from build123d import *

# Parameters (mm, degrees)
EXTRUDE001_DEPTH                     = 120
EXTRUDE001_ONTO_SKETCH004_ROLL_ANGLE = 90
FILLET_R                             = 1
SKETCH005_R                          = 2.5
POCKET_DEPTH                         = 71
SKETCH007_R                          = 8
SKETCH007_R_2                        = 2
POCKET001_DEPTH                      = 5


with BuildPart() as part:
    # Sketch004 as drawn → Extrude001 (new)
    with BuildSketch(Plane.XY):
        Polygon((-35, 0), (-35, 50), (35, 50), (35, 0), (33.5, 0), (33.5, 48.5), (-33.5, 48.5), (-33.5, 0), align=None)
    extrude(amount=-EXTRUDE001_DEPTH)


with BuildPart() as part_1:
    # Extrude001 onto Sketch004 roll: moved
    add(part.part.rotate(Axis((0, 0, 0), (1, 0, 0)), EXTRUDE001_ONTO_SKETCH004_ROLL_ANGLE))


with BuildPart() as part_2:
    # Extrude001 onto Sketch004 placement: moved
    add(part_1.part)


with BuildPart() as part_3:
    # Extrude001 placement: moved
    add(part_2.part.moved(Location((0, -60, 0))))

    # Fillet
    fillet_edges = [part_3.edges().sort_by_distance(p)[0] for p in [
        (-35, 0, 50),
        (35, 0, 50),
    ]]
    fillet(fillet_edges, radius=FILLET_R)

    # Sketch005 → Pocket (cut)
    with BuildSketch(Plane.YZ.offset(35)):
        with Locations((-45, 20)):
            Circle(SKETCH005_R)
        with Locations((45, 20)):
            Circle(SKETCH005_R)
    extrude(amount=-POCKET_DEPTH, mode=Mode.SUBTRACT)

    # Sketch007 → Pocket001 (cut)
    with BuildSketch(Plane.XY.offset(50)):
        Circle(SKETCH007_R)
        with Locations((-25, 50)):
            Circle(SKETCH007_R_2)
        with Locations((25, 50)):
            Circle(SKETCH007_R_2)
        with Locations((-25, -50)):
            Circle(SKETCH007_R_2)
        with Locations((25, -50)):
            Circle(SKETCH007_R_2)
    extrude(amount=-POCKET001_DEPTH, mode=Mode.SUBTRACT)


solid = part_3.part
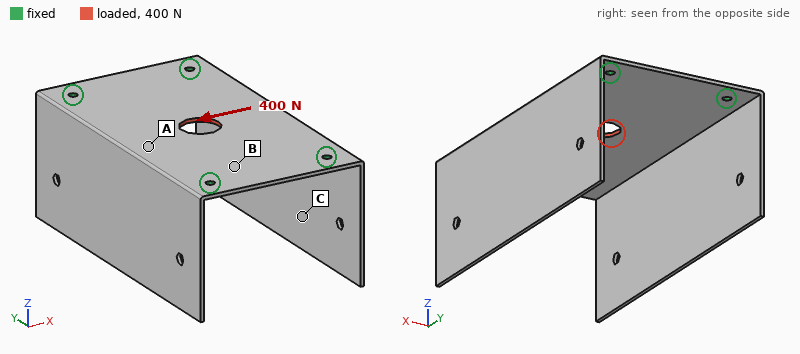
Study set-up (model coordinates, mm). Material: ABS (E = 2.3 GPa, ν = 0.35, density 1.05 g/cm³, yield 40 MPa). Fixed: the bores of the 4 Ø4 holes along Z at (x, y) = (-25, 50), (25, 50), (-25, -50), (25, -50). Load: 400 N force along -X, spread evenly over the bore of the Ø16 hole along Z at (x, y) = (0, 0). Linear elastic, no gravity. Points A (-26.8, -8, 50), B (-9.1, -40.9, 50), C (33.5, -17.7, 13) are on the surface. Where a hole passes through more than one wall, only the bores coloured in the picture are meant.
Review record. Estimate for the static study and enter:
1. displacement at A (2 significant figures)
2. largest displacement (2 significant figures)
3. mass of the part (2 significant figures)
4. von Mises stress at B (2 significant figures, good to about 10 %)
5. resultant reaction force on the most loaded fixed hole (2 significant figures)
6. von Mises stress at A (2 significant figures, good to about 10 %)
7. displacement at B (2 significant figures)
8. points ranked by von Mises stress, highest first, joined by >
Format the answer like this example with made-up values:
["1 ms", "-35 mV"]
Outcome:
["0.13 mm", "0.16 mm", "31 g", "3.7 MPa", "120 N", "2.6 MPa", "0.036 mm", "B > A > C"]
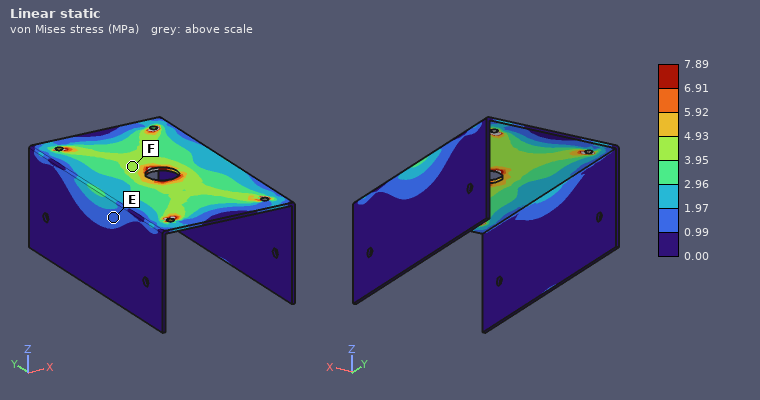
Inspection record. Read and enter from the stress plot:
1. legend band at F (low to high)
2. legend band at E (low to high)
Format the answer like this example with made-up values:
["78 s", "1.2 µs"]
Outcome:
["3.95 to 4.93 MPa", "0.99 to 1.97 MPa"]
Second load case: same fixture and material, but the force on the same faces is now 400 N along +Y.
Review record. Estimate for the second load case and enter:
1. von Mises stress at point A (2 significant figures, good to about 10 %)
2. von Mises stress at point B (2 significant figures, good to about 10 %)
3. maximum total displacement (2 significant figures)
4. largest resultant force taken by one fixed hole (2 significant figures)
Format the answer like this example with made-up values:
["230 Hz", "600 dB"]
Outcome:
["0.74 MPa", "1.8 MPa", "79 µm", "100 N"]
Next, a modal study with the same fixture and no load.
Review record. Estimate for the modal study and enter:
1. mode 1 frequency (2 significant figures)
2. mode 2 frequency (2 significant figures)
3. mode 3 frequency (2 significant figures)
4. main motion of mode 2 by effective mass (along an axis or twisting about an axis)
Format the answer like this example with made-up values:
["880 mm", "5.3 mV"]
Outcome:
["100 Hz", "110 Hz", "180 Hz", "along X"]
